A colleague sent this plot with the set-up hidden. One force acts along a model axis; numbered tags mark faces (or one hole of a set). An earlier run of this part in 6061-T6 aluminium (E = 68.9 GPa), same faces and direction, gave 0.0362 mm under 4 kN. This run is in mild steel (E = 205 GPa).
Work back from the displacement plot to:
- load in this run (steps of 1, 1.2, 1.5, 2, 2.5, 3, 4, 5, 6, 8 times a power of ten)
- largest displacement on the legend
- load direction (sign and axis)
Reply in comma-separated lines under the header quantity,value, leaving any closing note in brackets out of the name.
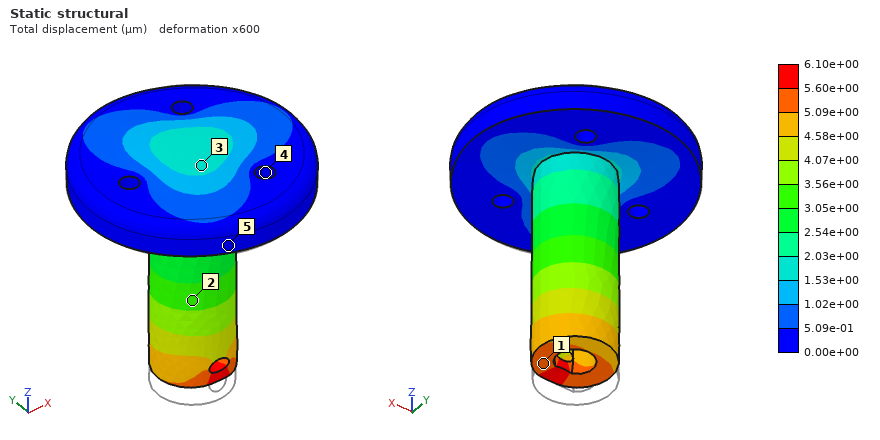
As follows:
quantity,value
load in this run,2 kN
largest displacement on the legend,6.10e+00 µm
load direction,+Z
